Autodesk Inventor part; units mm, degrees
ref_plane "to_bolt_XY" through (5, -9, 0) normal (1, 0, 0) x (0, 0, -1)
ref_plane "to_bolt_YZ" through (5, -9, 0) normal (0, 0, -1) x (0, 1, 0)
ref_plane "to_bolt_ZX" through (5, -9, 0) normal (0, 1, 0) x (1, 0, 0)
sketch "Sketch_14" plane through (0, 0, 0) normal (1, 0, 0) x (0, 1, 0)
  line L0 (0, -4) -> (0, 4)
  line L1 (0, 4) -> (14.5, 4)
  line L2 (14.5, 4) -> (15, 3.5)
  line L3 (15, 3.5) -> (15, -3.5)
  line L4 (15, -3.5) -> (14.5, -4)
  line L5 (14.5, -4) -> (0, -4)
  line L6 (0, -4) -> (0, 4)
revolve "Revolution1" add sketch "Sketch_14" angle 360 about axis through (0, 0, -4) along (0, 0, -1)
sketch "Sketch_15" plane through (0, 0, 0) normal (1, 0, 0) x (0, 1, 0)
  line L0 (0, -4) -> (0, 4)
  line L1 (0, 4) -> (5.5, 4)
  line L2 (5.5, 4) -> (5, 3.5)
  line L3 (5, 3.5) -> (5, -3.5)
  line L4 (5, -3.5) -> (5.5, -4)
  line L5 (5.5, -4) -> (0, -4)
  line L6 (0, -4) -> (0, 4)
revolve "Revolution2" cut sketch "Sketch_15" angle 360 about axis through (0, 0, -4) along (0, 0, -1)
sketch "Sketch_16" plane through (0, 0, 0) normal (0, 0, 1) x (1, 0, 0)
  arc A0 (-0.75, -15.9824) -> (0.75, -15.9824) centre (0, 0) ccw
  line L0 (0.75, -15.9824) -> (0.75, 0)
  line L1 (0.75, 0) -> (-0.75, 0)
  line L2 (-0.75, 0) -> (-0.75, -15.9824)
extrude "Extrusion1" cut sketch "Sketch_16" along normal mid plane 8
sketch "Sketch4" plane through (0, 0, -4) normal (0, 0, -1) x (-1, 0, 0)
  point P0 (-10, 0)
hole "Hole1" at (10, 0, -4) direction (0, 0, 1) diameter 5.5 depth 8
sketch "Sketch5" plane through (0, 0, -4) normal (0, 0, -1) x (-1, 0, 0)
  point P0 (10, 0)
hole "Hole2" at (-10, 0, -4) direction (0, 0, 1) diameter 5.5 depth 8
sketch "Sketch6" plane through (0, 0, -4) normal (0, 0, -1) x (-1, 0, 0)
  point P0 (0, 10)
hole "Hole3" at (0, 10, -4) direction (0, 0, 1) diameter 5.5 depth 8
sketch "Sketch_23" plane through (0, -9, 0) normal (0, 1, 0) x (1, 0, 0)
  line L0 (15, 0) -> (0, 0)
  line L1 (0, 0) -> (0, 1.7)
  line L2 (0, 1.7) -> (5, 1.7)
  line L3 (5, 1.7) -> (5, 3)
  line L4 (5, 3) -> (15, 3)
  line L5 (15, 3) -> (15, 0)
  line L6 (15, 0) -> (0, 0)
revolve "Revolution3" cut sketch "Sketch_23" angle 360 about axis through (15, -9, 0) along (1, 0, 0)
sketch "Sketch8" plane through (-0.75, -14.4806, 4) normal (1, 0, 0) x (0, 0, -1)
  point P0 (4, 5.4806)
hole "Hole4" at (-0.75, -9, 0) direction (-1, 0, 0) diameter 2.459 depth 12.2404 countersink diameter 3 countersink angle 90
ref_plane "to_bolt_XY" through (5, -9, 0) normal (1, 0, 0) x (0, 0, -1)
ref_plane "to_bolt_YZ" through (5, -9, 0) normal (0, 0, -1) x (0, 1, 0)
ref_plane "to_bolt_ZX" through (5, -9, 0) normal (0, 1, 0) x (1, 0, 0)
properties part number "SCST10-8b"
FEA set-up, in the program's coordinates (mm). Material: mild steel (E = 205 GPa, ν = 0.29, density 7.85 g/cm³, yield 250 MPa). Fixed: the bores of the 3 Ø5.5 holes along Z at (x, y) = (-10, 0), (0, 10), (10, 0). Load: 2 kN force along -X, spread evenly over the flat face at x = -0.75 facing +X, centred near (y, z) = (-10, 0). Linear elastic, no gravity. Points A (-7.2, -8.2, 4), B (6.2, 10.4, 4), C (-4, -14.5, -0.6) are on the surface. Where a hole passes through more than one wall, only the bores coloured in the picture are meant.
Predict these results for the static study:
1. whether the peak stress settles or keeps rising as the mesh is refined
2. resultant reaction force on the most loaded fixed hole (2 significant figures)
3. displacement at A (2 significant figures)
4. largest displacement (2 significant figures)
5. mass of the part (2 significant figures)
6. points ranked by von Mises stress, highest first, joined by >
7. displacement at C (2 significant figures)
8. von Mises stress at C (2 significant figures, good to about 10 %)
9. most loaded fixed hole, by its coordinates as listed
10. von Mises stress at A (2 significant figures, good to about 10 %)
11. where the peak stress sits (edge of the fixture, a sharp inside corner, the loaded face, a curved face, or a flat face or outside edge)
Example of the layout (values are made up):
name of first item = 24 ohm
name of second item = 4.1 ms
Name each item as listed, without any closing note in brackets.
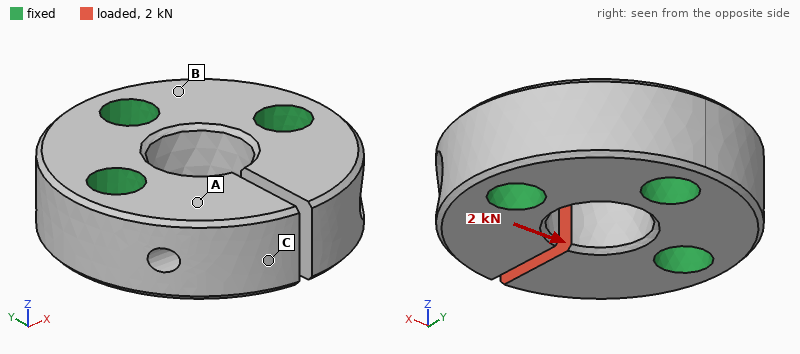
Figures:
whether the peak stress settles or keeps rising as the mesh is refined = keeps rising
resultant reaction force on the most loaded fixed hole = 2.1 kN
displacement at A = 5.9 µm
largest displacement = 17 µm
mass of the part = 32 g
points ranked by von Mises stress, highest first, joined by > = A > C > B
displacement at C = 14 µm
von Mises stress at C = 31 MPa
most loaded fixed hole, by its coordinates as listed = (-10, 0)
von Mises stress at A = 56 MPa
where the peak stress sits = edge of the fixture
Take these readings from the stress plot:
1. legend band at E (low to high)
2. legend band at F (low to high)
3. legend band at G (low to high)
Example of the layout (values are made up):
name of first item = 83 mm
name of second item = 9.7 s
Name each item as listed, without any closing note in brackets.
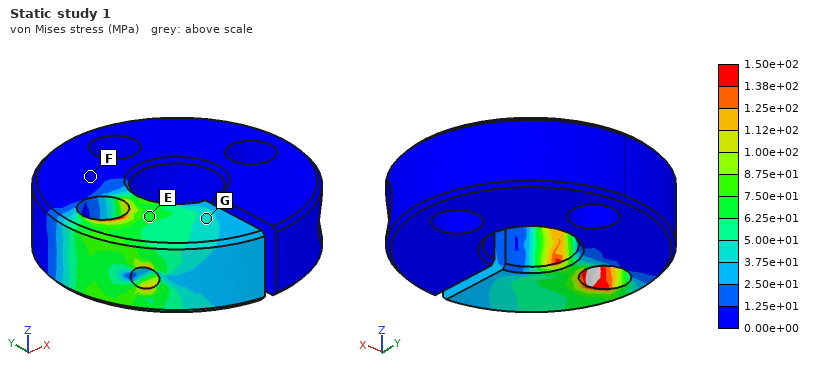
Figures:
legend band at E = 6.25e+01 to 7.50e+01 MPa
legend band at F = 0.00e+00 to 1.25e+01 MPa
legend band at G = 3.75e+01 to 5.00e+01 MPa
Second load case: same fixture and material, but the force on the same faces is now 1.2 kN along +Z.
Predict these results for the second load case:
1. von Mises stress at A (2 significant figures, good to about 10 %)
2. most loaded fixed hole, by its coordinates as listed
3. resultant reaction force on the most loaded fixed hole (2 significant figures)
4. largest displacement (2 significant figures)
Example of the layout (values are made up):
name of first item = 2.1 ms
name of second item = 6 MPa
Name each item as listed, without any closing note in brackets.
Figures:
von Mises stress at A = 72 MPa
most loaded fixed hole, by its coordinates as listed = (-10, 0)
resultant reaction force on the most loaded fixed hole = 1.2 kN
largest displacement = 17 µm
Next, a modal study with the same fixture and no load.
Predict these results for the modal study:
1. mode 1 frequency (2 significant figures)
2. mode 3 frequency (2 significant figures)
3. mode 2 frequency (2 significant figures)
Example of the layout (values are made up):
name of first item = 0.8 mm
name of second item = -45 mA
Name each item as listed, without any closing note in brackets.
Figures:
mode 1 frequency = 26 kHz
mode 3 frequency = 30 kHz
mode 2 frequency = 29 kHz
